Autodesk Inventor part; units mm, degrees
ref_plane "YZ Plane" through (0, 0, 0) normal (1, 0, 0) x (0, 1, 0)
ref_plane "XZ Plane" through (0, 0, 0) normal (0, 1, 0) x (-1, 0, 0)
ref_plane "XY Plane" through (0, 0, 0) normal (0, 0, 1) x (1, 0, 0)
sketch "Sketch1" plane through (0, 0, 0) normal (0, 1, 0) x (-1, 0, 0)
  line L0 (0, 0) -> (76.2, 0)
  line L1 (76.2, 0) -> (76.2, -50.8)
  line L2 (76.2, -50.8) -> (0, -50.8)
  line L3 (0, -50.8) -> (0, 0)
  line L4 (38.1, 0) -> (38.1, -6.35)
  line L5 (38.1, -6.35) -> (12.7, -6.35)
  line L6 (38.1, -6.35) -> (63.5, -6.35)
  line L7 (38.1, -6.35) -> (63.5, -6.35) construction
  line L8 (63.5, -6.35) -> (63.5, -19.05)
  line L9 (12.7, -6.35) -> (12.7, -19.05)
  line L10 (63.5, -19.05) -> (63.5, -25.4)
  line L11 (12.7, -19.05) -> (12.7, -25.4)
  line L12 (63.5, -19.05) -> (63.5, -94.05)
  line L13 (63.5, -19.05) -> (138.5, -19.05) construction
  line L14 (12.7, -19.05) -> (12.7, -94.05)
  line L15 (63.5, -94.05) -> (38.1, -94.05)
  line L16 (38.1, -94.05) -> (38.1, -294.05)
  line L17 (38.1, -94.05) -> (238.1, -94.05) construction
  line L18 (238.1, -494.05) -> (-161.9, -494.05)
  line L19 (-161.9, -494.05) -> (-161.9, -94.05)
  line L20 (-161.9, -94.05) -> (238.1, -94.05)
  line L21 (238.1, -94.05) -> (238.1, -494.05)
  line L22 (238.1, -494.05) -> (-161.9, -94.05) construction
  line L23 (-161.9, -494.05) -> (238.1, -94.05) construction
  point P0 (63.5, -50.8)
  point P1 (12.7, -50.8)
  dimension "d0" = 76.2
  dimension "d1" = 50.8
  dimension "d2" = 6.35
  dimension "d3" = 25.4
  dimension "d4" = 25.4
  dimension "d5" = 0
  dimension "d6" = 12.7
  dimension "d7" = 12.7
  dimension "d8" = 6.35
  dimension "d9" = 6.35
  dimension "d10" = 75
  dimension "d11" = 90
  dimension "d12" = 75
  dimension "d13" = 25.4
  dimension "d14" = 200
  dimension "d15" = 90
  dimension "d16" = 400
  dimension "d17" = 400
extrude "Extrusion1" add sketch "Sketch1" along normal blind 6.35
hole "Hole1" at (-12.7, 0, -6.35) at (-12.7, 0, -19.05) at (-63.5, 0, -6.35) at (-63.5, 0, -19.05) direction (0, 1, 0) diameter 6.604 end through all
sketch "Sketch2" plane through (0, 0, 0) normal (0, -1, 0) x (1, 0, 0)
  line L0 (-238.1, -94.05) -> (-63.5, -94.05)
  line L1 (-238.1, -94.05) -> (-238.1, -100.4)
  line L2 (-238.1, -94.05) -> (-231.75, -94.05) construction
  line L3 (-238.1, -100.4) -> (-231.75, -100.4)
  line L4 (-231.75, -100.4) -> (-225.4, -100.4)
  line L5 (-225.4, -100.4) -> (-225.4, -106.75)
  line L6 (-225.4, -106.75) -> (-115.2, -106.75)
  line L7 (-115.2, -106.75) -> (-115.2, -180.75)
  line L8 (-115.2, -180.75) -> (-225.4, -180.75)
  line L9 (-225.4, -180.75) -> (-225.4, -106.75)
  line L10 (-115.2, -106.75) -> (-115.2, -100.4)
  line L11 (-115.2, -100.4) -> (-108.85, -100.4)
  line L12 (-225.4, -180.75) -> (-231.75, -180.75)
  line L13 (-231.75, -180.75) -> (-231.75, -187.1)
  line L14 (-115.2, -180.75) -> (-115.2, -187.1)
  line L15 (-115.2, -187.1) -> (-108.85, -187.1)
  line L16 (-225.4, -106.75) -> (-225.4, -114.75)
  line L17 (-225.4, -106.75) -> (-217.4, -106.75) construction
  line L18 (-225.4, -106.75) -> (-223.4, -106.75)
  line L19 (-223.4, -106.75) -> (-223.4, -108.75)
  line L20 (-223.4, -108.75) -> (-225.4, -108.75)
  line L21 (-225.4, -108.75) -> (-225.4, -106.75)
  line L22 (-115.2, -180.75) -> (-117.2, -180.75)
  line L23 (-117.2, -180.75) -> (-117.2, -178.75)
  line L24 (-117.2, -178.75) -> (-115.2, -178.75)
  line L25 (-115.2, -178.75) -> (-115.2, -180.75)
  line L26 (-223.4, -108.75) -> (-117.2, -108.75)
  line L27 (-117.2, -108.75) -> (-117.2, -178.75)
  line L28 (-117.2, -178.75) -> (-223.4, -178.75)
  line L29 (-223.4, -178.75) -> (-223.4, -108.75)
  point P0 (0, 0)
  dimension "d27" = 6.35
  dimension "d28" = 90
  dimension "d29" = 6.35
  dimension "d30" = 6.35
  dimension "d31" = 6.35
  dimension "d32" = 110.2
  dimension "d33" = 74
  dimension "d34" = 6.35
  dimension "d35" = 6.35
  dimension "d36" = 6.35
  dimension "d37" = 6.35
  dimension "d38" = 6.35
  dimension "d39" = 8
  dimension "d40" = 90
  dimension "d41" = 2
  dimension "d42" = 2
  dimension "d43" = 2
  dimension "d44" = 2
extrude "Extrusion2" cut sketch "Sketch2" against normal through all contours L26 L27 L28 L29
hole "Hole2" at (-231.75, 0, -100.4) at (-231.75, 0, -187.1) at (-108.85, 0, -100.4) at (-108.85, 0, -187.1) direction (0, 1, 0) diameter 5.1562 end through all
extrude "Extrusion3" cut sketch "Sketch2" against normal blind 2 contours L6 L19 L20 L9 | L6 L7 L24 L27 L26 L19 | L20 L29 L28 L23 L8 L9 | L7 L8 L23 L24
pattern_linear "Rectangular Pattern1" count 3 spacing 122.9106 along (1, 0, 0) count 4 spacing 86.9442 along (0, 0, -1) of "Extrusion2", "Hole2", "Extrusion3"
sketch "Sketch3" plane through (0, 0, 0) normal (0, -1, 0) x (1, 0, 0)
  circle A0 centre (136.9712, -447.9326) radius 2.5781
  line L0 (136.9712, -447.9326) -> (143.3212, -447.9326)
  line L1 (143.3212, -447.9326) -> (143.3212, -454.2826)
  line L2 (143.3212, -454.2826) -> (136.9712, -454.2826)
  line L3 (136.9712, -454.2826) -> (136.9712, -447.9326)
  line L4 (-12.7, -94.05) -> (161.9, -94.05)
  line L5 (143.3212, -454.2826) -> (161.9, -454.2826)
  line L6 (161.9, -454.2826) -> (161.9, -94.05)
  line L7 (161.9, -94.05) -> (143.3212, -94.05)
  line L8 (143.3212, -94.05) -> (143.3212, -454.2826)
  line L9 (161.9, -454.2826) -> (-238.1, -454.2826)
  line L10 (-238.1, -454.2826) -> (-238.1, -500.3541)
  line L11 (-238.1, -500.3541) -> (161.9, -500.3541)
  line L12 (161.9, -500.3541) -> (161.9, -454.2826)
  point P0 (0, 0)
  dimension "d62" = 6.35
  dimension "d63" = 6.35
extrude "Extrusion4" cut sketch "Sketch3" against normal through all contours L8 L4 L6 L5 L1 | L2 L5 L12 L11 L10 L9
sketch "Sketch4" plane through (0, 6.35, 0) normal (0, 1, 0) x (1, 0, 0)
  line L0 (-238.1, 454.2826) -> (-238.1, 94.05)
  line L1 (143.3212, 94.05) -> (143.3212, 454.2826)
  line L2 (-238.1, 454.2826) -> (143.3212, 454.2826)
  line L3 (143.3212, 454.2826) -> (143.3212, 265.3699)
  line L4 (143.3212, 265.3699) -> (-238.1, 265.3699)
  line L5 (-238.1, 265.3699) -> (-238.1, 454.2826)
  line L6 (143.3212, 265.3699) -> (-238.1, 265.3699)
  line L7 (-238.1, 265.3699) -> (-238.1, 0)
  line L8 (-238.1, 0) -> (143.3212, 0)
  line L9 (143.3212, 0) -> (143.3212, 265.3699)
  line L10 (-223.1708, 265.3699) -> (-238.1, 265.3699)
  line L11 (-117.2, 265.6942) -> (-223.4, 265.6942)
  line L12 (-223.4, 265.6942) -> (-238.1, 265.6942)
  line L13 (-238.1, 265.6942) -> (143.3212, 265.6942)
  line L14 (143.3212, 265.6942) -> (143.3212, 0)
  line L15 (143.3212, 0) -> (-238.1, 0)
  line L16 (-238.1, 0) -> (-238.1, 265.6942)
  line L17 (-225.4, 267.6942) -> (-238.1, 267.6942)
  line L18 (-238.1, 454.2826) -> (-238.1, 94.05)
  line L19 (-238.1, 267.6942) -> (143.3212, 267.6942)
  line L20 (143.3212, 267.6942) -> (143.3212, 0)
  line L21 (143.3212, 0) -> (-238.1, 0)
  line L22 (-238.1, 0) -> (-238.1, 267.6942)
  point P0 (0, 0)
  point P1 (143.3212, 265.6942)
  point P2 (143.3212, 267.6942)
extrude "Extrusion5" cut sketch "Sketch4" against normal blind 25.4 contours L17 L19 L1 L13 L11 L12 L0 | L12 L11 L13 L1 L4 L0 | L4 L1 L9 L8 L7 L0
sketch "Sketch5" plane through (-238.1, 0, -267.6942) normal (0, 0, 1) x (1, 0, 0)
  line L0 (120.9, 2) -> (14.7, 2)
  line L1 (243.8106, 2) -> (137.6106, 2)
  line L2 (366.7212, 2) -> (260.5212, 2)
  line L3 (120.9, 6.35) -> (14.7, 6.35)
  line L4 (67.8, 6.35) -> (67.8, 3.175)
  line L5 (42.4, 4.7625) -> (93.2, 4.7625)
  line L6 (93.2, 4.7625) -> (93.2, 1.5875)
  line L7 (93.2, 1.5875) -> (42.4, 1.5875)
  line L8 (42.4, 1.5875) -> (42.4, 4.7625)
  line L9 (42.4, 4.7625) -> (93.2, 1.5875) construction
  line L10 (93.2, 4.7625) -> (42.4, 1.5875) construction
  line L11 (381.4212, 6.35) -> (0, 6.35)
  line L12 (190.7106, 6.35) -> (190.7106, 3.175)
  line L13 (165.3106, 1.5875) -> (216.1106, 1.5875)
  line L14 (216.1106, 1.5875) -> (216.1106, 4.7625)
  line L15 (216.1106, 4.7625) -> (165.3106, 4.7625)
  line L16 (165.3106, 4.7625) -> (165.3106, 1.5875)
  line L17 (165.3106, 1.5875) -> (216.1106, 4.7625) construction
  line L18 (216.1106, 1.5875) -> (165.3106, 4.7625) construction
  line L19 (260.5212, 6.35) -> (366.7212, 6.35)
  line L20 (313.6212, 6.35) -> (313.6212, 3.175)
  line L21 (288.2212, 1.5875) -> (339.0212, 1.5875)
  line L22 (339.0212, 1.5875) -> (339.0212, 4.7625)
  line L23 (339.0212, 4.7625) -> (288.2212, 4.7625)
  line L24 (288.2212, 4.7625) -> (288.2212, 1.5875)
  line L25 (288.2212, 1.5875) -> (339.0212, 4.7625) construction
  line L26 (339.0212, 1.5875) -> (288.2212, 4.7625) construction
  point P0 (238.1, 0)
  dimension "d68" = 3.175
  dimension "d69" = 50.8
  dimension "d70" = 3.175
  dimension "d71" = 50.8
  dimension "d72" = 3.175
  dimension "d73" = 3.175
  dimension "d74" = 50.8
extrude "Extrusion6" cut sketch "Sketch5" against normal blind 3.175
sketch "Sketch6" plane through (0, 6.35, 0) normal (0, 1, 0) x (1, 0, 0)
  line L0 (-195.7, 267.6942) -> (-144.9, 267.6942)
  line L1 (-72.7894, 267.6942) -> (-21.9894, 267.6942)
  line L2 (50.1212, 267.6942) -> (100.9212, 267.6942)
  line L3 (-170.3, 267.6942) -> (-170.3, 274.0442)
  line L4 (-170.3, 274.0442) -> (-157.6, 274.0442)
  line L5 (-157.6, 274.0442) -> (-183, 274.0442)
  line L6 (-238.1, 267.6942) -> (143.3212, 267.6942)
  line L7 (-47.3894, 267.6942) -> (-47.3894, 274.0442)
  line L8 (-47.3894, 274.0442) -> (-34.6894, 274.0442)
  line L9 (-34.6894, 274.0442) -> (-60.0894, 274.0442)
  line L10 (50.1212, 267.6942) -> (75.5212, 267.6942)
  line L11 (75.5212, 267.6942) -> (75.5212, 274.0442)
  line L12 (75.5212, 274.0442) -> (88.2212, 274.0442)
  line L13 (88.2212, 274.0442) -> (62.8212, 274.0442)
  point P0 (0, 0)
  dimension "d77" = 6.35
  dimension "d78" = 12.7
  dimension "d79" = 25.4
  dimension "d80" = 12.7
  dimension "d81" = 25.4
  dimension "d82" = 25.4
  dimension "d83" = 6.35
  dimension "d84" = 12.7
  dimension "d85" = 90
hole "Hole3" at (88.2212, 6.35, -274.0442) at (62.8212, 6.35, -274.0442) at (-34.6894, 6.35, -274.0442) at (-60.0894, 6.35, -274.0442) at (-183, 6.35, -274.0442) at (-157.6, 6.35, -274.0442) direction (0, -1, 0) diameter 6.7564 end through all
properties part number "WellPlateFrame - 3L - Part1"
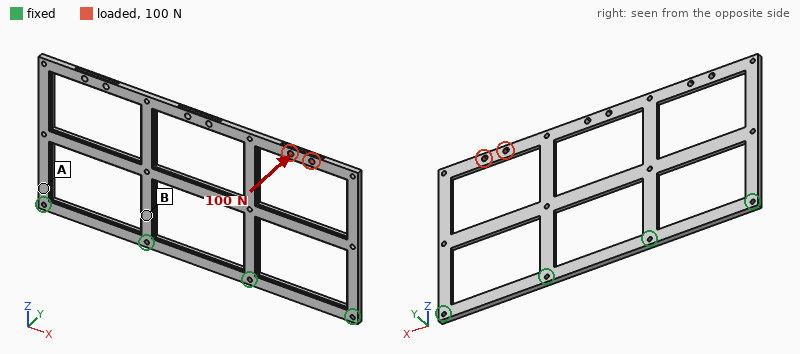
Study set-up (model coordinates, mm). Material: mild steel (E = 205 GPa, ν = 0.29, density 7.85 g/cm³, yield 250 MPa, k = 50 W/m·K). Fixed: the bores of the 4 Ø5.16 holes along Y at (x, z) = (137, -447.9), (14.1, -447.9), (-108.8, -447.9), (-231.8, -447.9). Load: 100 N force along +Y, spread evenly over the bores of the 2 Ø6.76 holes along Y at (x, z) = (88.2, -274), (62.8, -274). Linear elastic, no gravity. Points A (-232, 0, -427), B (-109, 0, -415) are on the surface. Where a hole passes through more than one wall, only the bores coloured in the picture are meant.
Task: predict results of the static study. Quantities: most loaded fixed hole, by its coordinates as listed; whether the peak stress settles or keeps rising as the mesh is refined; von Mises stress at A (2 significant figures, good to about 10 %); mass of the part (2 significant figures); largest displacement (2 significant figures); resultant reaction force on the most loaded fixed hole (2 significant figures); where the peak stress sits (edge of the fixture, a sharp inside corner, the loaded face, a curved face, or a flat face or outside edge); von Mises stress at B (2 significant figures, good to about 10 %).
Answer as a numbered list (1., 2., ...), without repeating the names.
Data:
1. (137, -447.9)
2. keeps rising
3. 17 MPa
4. 1.2 kg
5. 1.1 mm
6. 48 N
7. edge of the fixture
8. 30 MPa
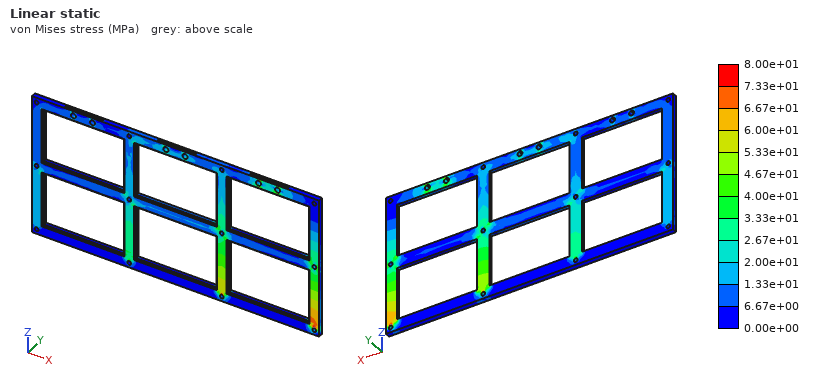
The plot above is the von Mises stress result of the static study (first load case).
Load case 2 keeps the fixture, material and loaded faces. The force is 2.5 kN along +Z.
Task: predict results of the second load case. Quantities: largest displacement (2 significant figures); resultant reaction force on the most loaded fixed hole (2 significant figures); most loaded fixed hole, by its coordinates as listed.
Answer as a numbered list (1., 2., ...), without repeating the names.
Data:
1. 0.17 mm
2. 1.4 kN
3. (14.1, -447.9)
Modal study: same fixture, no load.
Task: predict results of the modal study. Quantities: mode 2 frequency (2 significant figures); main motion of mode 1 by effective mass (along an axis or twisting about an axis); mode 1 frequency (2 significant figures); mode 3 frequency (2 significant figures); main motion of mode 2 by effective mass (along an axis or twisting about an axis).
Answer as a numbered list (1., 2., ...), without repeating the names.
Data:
1. 170 Hz
2. along Y
3. 100 Hz
4. 310 Hz
5. twisting about Z
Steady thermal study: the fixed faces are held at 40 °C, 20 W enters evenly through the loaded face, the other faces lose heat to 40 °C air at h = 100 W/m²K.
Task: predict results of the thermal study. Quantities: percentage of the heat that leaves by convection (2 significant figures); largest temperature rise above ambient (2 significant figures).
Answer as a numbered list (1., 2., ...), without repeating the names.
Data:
1. 100 %
2. 60 K
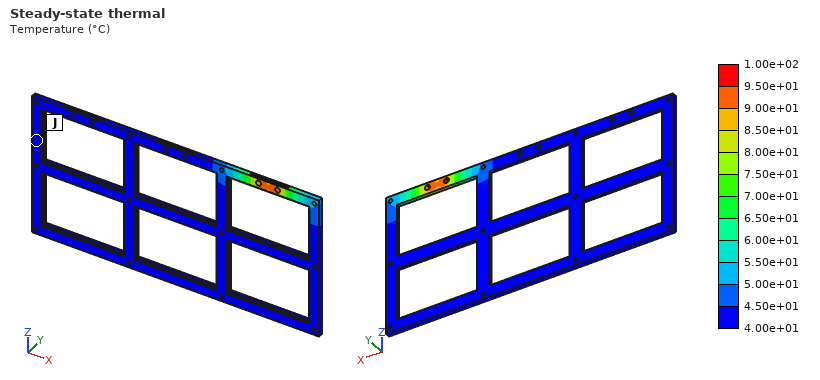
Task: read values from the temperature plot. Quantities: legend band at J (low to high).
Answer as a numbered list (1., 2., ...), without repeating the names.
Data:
1. 4.00e+01 to 4.50e+01 °C
